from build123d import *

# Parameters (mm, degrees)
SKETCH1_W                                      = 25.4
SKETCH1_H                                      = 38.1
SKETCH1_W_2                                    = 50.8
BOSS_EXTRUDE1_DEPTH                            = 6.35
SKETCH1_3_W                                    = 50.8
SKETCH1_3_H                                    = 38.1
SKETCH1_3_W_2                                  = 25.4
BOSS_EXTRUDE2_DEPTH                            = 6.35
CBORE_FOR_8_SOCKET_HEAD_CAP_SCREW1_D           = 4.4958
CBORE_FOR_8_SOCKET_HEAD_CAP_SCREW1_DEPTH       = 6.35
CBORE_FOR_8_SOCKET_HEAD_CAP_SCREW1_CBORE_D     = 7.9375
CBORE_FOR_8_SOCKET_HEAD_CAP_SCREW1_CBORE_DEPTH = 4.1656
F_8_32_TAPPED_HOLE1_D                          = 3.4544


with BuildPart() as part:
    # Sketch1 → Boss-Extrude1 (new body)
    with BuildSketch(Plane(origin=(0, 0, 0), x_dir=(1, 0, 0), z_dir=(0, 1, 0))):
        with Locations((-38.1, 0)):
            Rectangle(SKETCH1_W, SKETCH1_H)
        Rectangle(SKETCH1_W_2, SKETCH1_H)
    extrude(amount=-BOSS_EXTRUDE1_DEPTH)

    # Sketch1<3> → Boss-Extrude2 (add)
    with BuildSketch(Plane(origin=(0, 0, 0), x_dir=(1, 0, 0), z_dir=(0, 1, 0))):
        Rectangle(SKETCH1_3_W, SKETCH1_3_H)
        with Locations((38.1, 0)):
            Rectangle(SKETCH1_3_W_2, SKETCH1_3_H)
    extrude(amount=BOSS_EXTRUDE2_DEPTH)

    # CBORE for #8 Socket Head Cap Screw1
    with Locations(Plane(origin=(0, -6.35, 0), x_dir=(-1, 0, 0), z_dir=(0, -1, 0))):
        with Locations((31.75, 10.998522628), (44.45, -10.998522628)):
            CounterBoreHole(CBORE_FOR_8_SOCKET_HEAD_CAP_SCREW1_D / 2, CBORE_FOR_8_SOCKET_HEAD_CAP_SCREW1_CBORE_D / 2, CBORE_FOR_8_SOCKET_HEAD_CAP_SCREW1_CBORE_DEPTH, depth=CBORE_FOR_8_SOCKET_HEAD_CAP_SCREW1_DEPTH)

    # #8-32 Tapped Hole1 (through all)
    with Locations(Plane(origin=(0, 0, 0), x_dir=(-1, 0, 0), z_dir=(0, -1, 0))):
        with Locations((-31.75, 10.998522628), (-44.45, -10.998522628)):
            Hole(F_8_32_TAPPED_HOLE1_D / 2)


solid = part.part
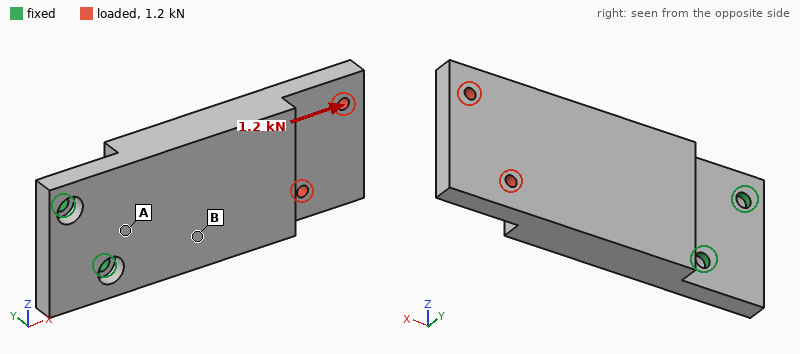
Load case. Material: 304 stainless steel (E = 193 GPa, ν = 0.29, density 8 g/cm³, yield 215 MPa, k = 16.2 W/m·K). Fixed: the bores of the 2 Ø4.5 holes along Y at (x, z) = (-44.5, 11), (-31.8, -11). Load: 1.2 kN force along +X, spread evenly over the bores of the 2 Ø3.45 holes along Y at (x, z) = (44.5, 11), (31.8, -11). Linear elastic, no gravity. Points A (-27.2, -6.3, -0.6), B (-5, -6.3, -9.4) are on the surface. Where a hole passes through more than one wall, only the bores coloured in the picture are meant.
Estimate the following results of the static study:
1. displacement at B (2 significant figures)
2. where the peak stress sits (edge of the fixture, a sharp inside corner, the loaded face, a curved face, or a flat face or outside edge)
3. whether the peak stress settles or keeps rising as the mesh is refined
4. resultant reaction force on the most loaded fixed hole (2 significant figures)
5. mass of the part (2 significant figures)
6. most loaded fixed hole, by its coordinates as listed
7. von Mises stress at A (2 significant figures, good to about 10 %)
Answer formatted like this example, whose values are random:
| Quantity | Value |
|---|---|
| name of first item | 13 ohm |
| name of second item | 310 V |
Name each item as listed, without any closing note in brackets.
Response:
| Quantity | Value |
|---|---|
| displacement at B | 27 µm |
| where the peak stress sits | edge of the fixture |
| whether the peak stress settles or keeps rising as the mesh is refined | keeps rising |
| resultant reaction force on the most loaded fixed hole | 670 N |
| mass of the part | 290 g |
| most loaded fixed hole, by its coordinates as listed | (-31.8, -11) |
| von Mises stress at A | 25 MPa |
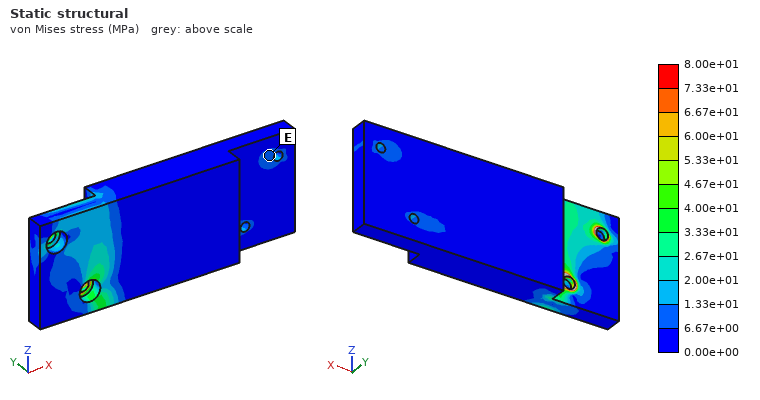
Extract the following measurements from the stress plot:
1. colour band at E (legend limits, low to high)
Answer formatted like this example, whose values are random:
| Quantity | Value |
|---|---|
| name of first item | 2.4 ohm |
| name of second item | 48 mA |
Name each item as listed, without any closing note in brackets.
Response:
| Quantity | Value |
|---|---|
| colour band at E | 6.67e+00 to 1.33e+01 MPa |
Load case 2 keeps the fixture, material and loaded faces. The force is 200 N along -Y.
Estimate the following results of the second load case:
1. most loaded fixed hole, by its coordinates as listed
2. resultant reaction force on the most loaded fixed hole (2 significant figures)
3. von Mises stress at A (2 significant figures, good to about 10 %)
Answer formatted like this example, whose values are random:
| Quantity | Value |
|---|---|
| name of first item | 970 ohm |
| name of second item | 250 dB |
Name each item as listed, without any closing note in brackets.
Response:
| Quantity | Value |
|---|---|
| most loaded fixed hole, by its coordinates as listed | (-31.8, -11) |
| resultant reaction force on the most loaded fixed hole | 380 N |
| von Mises stress at A | 55 MPa |
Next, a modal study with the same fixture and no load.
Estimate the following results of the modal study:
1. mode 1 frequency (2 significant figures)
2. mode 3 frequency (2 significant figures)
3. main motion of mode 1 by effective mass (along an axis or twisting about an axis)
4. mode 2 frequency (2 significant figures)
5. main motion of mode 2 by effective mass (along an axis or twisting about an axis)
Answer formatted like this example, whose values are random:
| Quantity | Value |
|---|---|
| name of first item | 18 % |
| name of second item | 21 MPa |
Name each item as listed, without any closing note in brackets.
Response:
| Quantity | Value |
|---|---|
| mode 1 frequency | 520 Hz |
| mode 3 frequency | 3600 Hz |
| main motion of mode 1 by effective mass | along Y |
| mode 2 frequency | 2500 Hz |
| main motion of mode 2 by effective mass | along Z |
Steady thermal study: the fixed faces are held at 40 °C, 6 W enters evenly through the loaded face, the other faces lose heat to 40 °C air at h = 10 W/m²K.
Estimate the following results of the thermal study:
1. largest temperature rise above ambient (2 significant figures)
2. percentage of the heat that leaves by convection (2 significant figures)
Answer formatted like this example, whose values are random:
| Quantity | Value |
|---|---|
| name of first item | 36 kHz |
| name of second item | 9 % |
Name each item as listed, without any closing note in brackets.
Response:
| Quantity | Value |
|---|---|
| largest temperature rise above ambient | 67 K |
| percentage of the heat that leaves by convection | 50 % |
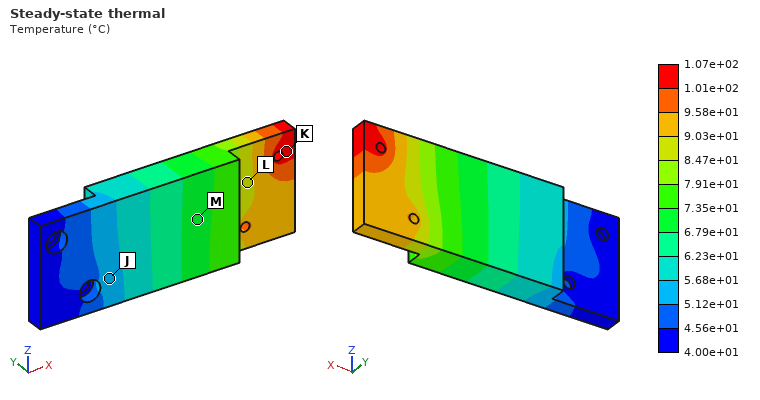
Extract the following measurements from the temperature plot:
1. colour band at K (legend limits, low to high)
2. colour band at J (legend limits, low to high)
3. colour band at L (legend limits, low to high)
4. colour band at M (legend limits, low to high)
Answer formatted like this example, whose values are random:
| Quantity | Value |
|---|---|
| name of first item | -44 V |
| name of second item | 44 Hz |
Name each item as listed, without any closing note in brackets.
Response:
| Quantity | Value |
|---|---|
| colour band at K | 1.01e+02 to 1.07e+02 °C |
| colour band at J | 5.12e+01 to 5.68e+01 °C |
| colour band at L | 8.47e+01 to 9.03e+01 °C |
| colour band at M | 6.79e+01 to 7.35e+01 °C |
